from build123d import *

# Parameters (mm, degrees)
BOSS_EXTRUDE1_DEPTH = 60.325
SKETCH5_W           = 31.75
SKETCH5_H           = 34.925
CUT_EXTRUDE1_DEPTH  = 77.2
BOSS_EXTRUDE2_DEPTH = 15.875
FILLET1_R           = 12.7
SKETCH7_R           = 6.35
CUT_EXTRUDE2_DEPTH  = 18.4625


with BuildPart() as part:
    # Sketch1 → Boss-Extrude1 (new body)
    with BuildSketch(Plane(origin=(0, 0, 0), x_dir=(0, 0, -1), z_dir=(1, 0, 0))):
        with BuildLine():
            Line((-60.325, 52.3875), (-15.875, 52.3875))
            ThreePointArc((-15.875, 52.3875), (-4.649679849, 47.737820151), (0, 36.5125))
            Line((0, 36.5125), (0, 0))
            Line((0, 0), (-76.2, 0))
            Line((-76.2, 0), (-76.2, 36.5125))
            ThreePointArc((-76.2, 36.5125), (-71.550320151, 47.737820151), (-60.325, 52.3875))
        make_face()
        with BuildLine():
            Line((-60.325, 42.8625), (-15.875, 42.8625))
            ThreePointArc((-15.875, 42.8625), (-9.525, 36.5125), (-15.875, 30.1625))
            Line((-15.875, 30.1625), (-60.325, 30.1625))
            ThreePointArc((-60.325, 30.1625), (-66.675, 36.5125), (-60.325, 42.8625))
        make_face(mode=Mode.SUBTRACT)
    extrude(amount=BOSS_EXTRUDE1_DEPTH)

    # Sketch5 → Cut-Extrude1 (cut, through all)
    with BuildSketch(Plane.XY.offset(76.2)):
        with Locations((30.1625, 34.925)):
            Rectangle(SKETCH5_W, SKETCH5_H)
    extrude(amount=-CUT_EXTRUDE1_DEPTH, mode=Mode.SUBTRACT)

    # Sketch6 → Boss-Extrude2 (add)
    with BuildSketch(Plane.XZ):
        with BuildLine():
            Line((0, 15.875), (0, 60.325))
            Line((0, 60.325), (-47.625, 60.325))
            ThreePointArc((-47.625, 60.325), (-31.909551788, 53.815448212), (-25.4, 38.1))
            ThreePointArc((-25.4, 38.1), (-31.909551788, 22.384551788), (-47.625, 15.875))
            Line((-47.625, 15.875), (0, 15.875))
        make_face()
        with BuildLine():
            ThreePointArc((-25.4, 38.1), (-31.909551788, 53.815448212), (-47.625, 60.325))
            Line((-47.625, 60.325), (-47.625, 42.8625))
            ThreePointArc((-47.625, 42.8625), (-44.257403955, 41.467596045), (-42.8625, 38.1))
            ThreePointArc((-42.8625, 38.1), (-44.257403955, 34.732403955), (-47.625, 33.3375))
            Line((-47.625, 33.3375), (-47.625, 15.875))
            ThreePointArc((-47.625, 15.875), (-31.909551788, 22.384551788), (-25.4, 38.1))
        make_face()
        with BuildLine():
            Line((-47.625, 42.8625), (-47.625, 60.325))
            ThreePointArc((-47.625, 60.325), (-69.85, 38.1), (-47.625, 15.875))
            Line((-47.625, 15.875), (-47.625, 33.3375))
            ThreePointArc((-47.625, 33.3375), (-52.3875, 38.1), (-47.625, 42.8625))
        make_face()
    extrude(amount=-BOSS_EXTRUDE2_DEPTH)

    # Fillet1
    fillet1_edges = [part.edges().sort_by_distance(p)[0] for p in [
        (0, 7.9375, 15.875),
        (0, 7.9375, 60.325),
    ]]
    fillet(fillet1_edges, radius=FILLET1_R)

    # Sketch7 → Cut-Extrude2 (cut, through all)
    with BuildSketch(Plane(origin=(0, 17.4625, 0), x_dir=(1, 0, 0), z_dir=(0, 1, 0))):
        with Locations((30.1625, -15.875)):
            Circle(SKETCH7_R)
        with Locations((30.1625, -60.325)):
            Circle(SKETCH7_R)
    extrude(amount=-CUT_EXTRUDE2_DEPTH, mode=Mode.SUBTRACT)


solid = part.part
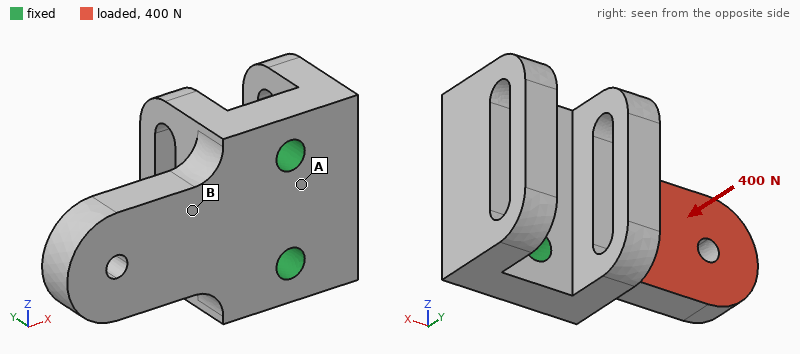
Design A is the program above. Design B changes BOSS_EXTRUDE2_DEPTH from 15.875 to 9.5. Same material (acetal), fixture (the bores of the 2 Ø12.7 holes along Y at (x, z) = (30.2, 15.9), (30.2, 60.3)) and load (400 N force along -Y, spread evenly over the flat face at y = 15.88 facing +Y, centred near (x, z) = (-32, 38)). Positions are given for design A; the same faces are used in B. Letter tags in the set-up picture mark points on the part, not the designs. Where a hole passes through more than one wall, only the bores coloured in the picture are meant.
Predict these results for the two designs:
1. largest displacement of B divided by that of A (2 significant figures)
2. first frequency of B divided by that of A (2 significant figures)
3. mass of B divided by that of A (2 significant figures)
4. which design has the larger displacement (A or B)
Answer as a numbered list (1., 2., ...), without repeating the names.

1. 2.8
2. 0.80
3. 0.89
4. B
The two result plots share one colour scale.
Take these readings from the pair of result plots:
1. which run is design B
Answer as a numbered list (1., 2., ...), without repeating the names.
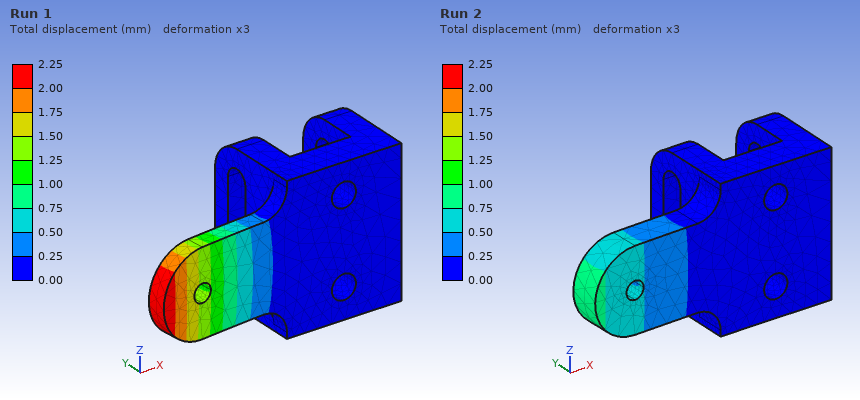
1. Run 1
